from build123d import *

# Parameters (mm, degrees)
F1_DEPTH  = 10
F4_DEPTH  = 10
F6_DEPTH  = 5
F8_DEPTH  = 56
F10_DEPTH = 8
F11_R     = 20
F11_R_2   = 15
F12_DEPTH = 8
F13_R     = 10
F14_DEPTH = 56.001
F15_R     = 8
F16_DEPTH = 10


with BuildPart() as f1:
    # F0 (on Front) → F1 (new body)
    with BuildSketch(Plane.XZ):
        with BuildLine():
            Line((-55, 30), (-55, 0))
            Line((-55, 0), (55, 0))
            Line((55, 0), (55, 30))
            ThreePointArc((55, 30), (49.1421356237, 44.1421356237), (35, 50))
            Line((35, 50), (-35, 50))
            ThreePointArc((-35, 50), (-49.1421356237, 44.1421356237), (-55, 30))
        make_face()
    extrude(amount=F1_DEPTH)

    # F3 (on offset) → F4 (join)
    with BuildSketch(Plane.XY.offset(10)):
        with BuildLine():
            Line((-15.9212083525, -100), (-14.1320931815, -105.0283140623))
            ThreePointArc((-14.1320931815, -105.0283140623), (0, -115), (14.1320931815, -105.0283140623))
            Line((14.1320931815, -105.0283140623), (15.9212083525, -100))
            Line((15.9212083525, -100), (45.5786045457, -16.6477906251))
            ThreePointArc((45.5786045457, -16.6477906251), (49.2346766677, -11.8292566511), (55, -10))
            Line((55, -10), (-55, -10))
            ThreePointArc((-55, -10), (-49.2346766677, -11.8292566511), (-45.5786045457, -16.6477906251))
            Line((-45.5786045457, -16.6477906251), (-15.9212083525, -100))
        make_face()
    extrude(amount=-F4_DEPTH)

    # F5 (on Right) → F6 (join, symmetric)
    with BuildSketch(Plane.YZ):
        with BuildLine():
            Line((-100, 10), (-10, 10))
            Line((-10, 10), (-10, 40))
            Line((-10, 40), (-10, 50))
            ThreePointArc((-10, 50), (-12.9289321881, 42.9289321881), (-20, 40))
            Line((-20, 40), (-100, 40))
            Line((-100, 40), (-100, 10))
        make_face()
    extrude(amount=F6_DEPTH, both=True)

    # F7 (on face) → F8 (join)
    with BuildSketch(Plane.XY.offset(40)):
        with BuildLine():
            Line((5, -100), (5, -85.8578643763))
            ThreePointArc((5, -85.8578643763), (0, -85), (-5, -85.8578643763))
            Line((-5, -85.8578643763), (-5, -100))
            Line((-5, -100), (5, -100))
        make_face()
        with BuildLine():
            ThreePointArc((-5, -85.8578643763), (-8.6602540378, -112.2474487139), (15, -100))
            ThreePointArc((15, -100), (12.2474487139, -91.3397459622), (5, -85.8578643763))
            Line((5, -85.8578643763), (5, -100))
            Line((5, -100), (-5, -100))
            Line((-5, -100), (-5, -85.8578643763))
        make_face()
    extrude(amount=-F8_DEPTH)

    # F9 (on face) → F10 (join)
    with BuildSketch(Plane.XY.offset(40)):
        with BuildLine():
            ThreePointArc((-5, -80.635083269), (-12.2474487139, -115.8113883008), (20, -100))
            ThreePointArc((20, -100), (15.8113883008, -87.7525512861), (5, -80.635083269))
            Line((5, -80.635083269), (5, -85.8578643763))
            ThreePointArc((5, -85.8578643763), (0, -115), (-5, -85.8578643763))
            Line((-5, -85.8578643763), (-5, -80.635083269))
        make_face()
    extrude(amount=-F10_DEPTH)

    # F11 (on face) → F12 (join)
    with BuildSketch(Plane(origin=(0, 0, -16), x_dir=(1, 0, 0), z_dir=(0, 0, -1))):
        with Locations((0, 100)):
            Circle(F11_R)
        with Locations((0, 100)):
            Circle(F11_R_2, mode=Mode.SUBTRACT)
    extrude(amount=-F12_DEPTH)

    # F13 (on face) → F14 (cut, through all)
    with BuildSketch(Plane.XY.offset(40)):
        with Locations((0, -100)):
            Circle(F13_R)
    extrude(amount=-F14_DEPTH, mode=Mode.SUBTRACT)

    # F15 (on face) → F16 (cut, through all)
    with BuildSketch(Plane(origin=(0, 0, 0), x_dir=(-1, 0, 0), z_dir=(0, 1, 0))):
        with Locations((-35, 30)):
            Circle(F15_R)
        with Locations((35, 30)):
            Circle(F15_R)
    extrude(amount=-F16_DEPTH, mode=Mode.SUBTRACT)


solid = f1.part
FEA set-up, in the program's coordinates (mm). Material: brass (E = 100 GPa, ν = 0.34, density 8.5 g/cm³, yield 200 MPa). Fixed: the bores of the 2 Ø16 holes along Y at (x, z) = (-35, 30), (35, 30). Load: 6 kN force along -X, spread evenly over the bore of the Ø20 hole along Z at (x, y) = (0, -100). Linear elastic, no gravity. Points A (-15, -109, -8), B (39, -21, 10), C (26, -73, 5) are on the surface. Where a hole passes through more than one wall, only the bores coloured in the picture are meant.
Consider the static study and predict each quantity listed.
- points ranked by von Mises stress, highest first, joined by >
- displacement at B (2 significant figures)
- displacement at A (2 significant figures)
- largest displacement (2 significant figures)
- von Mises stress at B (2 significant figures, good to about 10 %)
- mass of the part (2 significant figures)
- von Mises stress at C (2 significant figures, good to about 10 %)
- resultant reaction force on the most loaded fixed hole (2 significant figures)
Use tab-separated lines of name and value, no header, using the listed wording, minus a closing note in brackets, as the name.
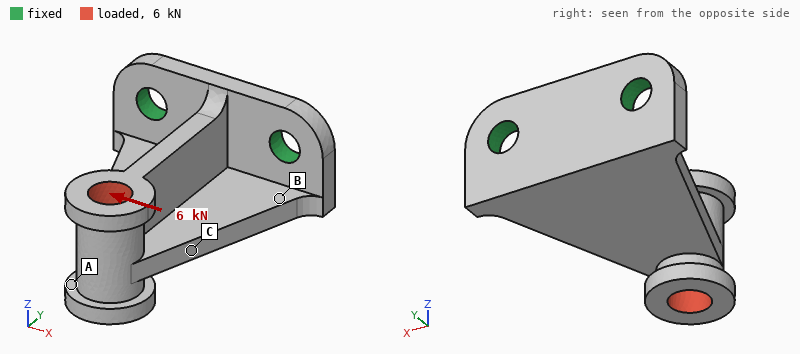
points ranked by von Mises stress, highest first, joined by >	B > C > A
displacement at B	0.060 mm
displacement at A	0.18 mm
largest displacement	0.34 mm
von Mises stress at B	77 MPa
mass of the part	1.3 kg
von Mises stress at C	45 MPa
resultant reaction force on the most loaded fixed hole	8.7 kN
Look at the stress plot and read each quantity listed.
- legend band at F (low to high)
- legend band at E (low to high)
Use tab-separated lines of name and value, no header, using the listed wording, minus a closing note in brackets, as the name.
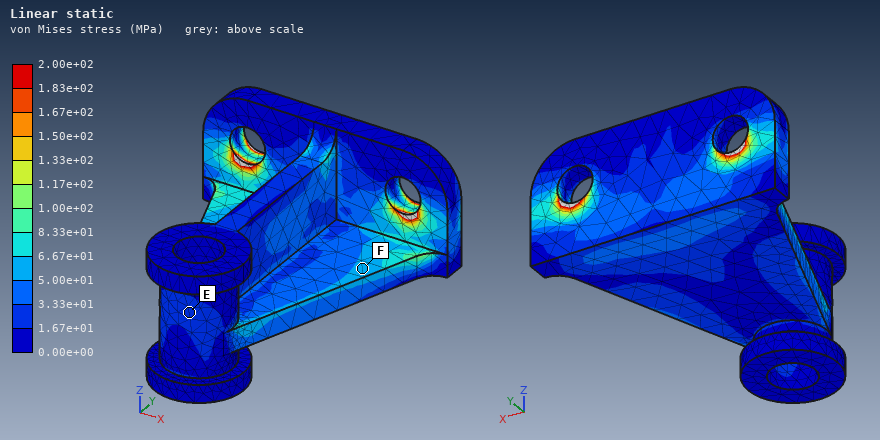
legend band at F	5.00e+01 to 6.67e+01 MPa
legend band at E	1.67e+01 to 3.33e+01 MPa
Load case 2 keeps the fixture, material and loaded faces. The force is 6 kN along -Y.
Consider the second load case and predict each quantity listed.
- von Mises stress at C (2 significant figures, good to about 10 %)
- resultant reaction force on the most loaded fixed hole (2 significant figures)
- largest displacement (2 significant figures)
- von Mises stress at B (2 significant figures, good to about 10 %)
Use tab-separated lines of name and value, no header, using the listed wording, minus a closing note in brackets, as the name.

von Mises stress at C	8.4 MPa
resultant reaction force on the most loaded fixed hole	3.0 kN
largest displacement	73 µm
von Mises stress at B	18 MPa
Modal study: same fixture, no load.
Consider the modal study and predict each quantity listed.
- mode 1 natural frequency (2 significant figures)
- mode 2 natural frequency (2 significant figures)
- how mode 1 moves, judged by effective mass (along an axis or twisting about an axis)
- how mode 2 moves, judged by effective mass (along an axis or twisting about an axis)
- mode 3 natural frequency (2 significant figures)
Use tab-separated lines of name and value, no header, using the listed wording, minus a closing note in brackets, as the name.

mode 1 natural frequency	710 Hz
mode 2 natural frequency	1300 Hz
how mode 1 moves, judged by effective mass	along Z
how mode 2 moves, judged by effective mass	along X
mode 3 natural frequency	1900 Hz
